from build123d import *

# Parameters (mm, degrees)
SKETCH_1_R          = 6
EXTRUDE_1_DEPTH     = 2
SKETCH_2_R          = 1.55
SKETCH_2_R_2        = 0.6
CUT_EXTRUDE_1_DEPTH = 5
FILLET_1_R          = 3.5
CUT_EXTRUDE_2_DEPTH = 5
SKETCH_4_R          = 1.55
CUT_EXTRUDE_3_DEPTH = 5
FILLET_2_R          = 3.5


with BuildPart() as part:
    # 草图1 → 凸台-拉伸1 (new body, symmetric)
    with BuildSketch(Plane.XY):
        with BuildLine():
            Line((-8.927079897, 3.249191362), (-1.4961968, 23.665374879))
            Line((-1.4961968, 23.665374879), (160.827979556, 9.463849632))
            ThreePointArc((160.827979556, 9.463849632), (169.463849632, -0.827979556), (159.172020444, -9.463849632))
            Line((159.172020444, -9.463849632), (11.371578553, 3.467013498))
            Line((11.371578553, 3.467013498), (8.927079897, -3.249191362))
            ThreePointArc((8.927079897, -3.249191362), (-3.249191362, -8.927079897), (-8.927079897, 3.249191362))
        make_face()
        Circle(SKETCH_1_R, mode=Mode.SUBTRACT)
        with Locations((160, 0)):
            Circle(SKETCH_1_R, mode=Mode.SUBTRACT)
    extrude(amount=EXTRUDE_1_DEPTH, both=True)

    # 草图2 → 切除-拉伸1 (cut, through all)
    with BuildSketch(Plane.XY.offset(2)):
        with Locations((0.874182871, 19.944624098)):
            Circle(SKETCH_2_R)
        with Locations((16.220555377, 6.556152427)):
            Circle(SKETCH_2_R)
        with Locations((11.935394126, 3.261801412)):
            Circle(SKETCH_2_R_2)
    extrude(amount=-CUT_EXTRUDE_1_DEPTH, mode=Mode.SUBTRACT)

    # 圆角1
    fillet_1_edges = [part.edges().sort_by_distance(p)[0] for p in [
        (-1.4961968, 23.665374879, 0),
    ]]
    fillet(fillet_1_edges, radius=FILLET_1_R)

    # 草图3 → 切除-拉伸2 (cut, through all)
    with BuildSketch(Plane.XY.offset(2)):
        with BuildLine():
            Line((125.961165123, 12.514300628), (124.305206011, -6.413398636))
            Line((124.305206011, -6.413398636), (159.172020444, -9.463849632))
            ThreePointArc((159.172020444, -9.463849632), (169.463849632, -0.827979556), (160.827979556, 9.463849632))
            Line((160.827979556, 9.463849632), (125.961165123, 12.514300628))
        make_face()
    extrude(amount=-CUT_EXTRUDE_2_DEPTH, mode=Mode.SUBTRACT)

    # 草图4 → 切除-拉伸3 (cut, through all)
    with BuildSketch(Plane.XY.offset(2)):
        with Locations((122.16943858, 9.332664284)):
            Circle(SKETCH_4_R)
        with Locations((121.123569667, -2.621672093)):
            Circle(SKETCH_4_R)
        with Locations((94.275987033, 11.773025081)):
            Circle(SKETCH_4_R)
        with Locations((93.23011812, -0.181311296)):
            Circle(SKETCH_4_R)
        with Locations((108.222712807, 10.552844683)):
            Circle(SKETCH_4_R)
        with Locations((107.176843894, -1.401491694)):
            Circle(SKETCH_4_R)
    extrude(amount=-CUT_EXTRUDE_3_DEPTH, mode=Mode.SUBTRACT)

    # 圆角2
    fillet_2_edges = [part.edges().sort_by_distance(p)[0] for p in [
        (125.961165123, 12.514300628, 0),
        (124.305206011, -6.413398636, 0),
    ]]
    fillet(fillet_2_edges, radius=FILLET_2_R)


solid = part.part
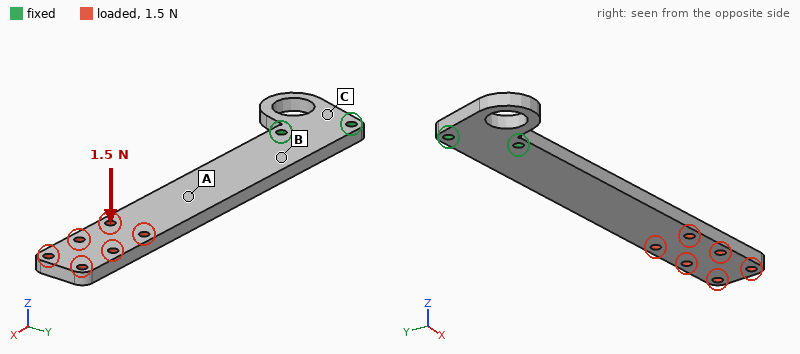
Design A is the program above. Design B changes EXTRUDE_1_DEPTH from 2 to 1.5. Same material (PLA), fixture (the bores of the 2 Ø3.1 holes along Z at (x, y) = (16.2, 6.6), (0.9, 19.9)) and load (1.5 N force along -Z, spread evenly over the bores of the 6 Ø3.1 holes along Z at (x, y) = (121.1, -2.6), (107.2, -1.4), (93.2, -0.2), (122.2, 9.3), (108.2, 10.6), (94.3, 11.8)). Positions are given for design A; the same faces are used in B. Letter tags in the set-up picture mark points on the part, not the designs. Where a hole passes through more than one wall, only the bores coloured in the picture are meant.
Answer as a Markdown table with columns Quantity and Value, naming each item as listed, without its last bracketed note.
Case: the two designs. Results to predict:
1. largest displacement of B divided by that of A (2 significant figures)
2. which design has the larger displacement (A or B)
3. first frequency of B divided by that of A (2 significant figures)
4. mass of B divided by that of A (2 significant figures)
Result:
| Quantity | Value |
|---|---|
| largest displacement of B divided by that of A | 2.3 |
| which design has the larger displacement | B |
| first frequency of B divided by that of A | 0.75 |
| mass of B divided by that of A | 0.75 |
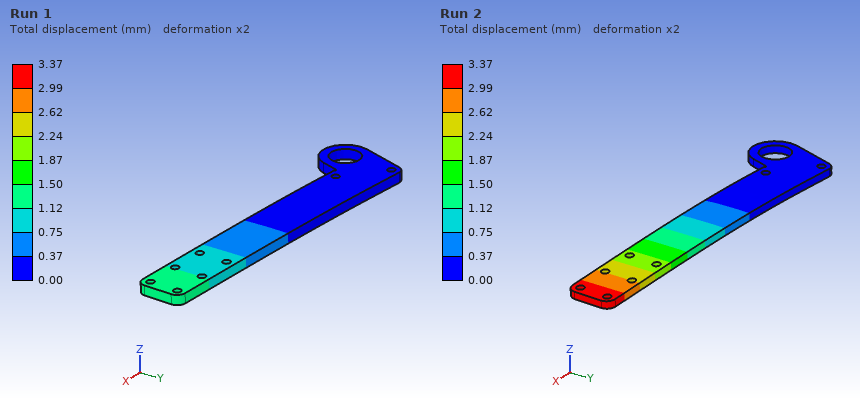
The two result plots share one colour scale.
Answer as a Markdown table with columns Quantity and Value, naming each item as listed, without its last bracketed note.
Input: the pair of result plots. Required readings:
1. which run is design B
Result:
| Quantity | Value |
|---|---|
| which run is design B | Run 2 |
